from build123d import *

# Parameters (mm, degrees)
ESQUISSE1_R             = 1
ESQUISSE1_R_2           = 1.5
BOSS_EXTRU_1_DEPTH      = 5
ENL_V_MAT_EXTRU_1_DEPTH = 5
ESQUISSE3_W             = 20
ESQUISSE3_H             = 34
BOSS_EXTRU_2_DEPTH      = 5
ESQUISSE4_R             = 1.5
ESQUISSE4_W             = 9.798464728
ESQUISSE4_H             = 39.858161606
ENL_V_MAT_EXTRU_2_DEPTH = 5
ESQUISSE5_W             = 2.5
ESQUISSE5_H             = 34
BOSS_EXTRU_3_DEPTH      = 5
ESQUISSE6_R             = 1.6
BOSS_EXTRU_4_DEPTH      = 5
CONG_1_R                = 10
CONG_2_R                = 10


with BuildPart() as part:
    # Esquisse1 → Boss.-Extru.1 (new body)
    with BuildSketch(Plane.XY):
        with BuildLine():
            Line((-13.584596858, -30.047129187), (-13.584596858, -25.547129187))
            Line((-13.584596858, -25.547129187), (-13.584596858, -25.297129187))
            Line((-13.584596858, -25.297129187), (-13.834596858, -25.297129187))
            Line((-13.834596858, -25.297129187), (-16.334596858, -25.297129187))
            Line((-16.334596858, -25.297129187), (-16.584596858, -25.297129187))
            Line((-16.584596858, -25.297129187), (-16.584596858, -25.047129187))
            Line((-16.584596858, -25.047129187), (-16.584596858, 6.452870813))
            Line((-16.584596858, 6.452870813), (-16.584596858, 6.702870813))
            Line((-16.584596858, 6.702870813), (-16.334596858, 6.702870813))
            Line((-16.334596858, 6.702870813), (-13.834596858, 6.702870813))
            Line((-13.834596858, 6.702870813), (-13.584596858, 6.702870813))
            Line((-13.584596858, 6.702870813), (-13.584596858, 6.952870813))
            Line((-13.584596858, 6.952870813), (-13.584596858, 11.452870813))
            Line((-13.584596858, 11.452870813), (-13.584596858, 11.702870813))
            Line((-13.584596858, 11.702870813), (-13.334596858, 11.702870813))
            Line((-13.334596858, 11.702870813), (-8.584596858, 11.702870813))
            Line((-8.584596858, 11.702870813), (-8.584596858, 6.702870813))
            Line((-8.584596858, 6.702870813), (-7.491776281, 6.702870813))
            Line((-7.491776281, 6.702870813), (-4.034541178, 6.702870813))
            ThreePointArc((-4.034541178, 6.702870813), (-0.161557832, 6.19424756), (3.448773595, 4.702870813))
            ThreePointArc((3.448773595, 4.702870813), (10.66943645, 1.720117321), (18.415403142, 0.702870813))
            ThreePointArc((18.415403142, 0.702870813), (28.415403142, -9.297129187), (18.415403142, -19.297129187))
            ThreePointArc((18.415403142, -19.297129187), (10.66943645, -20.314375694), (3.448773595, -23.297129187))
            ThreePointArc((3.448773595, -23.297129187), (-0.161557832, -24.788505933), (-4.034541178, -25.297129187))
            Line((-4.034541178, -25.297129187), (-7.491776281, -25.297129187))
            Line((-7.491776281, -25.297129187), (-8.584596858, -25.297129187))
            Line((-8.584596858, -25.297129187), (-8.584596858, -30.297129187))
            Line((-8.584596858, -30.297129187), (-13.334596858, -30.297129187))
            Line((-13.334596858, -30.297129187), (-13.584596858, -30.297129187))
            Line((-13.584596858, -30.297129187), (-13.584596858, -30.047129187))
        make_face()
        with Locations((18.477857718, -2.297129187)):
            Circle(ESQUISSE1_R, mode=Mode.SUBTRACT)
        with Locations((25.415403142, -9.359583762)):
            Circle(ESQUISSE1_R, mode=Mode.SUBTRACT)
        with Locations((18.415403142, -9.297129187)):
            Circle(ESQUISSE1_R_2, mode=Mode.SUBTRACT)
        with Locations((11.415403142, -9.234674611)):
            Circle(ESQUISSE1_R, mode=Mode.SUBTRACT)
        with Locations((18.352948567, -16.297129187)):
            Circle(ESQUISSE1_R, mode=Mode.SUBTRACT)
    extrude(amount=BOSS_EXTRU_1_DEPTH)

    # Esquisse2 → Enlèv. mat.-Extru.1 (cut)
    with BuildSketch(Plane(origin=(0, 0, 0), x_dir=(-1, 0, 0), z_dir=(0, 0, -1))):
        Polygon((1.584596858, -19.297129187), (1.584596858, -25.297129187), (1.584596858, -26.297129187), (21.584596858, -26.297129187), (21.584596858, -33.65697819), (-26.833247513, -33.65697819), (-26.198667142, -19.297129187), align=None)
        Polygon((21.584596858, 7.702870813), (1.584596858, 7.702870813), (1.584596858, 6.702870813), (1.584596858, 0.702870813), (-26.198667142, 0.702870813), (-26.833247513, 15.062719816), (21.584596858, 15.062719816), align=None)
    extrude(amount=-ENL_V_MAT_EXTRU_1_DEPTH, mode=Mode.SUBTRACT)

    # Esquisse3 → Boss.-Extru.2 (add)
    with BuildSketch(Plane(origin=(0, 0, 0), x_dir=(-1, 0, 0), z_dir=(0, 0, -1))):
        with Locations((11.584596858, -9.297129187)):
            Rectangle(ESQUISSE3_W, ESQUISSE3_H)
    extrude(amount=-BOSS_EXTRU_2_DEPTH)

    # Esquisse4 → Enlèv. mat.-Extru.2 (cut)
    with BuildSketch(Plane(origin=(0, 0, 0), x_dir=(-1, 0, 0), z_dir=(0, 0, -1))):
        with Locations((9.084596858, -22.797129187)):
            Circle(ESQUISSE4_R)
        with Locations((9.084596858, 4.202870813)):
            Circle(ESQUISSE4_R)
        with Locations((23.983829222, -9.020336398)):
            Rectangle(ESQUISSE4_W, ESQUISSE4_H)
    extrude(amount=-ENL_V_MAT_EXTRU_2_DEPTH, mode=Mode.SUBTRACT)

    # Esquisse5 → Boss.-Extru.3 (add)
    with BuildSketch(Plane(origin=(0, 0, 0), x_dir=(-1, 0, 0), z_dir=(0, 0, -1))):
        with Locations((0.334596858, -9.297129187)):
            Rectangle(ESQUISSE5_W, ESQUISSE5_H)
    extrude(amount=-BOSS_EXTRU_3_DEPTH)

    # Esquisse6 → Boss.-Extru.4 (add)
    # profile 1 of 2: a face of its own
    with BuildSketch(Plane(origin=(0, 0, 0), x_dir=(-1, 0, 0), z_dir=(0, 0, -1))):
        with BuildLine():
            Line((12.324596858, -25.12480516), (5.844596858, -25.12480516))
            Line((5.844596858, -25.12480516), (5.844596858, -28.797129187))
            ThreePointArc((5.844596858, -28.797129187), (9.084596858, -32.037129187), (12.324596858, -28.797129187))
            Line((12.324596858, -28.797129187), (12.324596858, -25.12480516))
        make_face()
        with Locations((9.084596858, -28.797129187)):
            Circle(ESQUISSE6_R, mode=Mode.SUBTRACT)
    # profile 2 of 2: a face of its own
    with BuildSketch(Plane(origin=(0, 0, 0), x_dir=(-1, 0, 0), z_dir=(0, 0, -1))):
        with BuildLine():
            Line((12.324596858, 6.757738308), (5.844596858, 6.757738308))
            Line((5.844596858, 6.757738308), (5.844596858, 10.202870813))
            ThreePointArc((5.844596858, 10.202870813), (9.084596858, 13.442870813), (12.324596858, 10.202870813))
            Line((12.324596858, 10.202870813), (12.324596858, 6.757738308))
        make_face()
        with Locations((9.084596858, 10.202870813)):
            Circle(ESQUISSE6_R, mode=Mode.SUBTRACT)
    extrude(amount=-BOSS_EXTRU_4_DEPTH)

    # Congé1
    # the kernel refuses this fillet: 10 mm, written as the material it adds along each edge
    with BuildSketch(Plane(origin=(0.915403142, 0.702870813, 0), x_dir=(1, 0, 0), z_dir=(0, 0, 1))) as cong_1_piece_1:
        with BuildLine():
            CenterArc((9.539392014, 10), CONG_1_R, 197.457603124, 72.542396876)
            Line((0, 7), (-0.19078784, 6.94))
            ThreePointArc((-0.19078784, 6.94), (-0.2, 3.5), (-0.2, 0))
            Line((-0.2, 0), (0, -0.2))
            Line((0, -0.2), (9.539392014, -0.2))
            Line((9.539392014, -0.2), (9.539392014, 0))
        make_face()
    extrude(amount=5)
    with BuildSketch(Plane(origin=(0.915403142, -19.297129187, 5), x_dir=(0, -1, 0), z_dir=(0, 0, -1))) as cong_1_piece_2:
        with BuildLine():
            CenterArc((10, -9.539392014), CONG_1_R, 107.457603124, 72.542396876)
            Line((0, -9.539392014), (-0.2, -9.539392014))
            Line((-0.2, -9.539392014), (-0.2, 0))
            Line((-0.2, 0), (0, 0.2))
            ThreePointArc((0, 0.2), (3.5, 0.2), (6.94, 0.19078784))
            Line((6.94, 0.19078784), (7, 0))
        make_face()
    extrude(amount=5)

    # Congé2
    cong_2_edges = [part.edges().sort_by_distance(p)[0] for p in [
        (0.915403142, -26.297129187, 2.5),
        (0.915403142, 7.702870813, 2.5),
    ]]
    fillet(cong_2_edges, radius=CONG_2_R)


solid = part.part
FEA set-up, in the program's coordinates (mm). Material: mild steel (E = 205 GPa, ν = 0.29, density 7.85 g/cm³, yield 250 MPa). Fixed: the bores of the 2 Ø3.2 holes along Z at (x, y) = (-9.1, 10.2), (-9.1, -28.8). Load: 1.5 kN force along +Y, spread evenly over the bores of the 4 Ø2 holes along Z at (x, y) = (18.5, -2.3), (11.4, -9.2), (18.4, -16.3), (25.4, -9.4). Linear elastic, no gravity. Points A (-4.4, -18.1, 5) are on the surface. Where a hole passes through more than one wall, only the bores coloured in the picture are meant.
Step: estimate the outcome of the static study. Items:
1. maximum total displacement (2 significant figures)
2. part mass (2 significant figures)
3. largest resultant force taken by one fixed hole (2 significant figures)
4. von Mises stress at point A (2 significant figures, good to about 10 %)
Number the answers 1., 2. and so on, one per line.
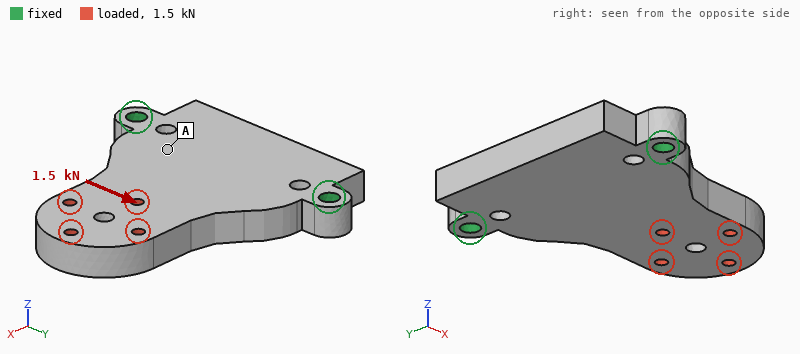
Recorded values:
1. 17 µm
2. 48 g
3. 1.4 kN
4. 16 MPa
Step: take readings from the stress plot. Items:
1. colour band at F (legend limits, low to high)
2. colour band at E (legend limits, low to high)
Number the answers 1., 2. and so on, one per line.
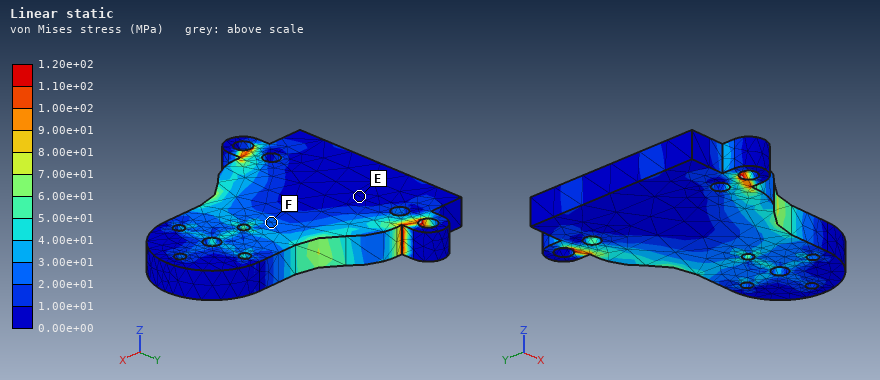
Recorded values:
1. 2.00e+01 to 3.00e+01 MPa
2. 0.00e+00 to 1.00e+01 MPa
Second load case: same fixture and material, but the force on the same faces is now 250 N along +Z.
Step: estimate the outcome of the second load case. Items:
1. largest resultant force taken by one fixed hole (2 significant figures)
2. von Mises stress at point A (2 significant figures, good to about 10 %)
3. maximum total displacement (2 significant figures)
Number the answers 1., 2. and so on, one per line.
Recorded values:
1. 130 N
2. 42 MPa
3. 92 µm
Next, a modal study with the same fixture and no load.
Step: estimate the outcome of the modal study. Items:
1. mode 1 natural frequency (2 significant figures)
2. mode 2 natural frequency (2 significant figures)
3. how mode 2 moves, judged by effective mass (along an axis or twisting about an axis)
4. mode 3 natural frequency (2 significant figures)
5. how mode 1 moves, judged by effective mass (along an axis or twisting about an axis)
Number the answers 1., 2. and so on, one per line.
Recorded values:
1. 2600 Hz
2. 12 kHz
3. along Z
4. 13 kHz
5. along Z
